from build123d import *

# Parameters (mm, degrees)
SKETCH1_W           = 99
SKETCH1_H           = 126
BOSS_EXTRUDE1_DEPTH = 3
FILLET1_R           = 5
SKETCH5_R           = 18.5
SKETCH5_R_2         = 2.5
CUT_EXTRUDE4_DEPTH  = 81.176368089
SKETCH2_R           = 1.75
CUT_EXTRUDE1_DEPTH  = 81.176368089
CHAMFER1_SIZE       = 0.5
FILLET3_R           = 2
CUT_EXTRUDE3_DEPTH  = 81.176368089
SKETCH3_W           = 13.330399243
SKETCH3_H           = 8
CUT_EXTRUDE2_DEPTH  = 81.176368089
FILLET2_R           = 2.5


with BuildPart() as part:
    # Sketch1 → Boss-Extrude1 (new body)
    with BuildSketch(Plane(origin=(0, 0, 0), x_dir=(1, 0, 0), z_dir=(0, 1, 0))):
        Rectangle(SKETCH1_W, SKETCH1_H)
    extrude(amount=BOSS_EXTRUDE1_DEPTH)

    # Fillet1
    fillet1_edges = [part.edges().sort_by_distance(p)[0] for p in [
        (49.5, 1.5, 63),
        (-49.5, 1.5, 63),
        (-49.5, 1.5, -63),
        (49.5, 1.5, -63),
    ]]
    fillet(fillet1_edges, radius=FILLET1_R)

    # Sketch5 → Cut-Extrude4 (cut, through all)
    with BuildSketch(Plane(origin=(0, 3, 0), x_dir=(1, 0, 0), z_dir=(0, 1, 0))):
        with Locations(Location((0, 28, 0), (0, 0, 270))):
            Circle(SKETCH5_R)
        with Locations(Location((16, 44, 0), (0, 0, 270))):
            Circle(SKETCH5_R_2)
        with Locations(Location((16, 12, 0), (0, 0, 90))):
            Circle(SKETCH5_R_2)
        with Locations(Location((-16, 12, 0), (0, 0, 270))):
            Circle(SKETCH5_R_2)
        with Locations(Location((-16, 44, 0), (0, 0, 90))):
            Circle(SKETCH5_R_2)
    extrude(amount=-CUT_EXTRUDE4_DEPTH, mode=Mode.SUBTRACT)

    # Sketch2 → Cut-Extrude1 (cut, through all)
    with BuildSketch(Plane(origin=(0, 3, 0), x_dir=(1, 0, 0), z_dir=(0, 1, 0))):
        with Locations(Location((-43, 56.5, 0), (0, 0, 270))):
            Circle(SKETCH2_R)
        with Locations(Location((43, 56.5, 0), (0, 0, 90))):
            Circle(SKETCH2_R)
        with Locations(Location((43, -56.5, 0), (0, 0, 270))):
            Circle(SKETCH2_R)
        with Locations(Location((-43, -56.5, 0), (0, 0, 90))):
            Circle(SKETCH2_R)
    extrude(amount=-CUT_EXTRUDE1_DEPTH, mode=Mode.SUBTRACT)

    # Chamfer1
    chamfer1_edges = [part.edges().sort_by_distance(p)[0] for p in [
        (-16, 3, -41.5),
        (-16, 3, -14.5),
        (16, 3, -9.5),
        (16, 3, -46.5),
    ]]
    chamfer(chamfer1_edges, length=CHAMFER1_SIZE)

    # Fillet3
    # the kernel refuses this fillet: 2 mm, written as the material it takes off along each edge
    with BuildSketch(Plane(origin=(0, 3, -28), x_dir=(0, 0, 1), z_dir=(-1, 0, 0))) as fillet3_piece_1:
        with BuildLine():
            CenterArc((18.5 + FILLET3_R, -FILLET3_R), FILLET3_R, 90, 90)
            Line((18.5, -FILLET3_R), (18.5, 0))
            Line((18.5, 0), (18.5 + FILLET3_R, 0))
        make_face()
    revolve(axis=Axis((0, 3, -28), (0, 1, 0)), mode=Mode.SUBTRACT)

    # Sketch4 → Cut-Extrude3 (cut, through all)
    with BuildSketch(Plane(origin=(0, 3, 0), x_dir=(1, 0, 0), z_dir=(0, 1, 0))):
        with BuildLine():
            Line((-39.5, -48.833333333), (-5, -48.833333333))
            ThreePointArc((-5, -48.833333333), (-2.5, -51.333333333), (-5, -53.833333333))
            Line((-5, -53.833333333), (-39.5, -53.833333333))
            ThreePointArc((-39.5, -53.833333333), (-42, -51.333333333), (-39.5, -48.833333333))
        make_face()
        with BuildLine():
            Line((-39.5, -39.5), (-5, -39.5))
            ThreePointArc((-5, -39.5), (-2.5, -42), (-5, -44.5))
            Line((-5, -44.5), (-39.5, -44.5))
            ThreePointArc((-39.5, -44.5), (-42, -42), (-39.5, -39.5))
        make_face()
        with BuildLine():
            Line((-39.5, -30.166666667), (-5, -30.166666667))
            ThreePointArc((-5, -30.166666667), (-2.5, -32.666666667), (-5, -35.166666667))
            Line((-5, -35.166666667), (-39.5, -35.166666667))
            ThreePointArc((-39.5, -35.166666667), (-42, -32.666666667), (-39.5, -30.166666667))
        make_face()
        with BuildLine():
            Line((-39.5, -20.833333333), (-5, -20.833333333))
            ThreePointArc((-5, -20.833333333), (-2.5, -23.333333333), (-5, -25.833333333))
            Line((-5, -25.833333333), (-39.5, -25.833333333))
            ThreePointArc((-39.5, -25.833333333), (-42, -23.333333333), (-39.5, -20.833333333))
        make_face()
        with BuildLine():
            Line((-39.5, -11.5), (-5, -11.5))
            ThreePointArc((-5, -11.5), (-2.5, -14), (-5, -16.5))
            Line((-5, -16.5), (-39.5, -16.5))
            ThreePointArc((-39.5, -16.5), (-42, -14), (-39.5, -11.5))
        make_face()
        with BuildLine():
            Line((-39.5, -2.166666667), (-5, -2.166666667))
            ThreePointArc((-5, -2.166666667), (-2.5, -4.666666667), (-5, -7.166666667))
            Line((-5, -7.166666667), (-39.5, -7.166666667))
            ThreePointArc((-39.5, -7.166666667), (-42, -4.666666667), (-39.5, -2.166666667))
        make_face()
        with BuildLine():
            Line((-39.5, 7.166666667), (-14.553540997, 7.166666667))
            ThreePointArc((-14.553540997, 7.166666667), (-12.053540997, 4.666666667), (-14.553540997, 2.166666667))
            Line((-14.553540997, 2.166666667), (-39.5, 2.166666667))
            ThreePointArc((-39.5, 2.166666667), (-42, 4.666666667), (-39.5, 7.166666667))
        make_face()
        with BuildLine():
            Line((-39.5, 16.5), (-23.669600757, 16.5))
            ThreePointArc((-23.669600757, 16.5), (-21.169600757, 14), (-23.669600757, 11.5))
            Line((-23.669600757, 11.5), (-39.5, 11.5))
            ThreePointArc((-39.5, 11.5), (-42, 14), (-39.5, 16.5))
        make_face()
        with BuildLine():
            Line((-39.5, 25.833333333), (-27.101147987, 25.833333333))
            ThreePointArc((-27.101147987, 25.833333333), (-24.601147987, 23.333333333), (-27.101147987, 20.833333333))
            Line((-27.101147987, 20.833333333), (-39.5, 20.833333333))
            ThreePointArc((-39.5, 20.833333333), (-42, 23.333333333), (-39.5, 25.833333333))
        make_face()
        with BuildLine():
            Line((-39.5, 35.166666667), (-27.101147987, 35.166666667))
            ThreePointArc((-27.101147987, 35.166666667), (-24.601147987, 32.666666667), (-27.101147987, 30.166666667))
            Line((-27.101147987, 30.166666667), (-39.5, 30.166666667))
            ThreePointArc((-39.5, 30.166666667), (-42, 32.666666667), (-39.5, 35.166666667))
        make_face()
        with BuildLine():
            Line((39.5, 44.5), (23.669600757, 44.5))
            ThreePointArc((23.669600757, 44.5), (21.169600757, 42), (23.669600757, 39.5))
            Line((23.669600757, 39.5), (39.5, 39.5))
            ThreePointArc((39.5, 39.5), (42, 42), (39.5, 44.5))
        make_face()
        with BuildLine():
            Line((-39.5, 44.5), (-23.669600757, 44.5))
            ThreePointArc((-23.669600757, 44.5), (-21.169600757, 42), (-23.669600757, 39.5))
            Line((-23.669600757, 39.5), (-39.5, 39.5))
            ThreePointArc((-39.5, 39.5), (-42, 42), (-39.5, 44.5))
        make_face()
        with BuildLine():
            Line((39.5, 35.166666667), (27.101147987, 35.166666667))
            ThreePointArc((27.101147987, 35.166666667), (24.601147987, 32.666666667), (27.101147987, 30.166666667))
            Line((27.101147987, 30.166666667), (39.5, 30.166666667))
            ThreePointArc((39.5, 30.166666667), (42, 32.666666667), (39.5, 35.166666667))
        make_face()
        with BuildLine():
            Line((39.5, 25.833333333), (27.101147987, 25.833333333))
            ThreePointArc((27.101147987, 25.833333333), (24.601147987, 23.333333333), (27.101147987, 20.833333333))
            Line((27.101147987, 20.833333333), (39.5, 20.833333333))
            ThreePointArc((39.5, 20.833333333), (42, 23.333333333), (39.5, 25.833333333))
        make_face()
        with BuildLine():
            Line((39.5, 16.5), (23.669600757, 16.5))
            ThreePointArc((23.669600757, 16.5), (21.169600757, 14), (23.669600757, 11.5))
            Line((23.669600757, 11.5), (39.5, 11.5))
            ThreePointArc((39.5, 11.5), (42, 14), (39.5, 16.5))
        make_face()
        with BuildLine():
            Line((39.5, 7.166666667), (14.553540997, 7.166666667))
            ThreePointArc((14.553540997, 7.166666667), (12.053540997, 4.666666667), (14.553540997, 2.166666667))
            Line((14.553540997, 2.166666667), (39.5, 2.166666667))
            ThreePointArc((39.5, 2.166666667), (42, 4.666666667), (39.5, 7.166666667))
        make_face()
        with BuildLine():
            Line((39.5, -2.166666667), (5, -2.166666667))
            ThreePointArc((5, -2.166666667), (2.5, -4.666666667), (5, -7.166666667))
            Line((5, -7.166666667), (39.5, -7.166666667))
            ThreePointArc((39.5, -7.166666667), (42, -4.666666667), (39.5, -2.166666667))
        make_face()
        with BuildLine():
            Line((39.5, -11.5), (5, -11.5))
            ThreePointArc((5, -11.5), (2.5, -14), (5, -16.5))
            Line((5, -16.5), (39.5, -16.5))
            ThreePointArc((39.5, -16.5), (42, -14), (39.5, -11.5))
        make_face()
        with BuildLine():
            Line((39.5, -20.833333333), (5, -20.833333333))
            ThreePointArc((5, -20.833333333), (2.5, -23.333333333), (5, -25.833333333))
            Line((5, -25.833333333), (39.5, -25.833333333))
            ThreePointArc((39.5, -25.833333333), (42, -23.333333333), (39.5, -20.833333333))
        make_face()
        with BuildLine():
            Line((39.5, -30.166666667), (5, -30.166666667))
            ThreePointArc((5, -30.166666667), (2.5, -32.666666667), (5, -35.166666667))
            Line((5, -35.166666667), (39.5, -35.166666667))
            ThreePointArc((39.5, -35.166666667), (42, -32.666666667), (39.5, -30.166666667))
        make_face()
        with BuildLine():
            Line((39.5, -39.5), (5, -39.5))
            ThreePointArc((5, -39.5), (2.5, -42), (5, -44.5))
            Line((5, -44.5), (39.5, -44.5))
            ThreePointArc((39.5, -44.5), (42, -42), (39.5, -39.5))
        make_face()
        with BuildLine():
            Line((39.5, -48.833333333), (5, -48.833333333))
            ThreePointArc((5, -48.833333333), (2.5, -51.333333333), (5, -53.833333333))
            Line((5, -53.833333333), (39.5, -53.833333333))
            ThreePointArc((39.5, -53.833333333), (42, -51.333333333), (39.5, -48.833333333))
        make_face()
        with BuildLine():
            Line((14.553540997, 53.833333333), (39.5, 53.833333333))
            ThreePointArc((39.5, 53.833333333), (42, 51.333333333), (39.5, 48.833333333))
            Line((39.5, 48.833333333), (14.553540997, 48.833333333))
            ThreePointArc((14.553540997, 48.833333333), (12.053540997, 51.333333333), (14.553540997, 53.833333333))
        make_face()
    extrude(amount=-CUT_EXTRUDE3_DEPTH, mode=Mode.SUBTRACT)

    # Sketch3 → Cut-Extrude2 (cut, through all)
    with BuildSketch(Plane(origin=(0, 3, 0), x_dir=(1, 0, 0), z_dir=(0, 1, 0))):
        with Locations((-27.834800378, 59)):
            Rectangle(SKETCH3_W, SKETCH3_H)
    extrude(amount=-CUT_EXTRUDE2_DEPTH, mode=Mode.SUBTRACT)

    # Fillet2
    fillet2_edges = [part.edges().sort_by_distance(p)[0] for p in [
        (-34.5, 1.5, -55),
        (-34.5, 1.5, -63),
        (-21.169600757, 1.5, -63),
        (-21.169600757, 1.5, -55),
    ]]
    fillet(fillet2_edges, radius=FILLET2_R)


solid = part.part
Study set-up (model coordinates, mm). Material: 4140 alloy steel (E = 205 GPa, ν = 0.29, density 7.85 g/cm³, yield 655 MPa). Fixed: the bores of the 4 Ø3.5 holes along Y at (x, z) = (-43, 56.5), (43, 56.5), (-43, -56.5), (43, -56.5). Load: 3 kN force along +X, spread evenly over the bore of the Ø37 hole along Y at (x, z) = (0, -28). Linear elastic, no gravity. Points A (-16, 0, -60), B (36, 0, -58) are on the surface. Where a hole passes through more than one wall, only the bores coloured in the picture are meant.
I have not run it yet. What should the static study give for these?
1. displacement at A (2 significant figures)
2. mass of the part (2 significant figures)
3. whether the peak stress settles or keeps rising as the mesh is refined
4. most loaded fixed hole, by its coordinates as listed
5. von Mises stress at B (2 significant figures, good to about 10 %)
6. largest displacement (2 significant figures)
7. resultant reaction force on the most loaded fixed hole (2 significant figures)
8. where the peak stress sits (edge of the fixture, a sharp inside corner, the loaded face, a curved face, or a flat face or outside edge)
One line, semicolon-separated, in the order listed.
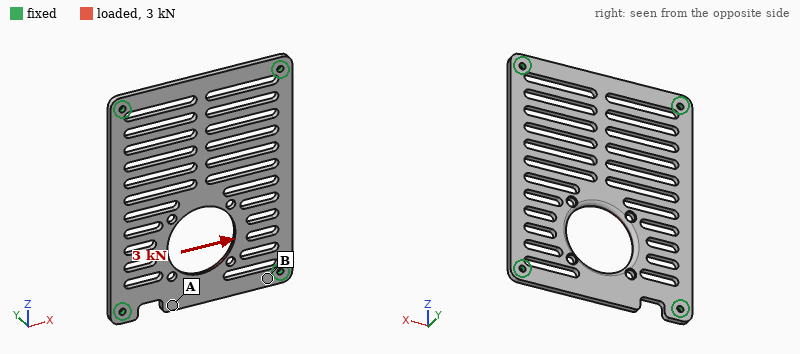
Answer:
8.5 µm; 180 g; keeps rising; (43, -56.5); 37 MPa; 43 µm; 1.6 kN; a sharp inside corner
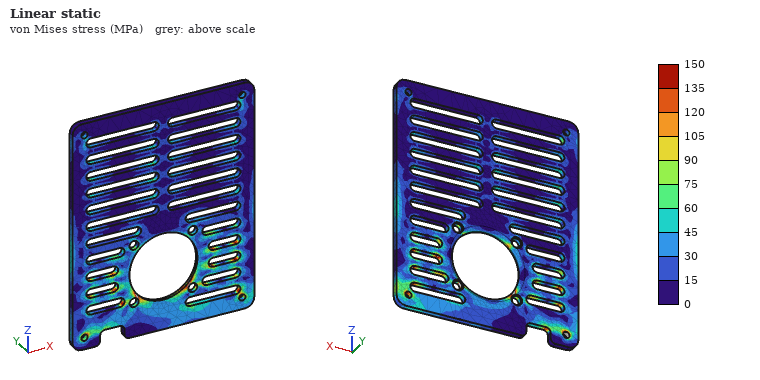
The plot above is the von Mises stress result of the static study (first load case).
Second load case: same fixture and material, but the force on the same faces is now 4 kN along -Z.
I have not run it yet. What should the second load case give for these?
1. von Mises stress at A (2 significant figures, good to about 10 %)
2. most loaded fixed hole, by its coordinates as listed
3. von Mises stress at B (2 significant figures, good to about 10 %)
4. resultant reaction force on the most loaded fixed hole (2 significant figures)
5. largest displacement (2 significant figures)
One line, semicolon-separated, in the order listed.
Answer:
29 MPa; (-43, -56.5); 57 MPa; 1.7 kN; 79 µm
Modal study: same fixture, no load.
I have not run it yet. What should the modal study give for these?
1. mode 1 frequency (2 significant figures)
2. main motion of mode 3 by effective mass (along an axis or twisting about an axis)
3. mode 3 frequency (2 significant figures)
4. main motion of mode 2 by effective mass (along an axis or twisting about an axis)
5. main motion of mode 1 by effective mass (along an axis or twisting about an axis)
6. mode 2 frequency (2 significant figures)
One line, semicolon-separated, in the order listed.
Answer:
740 Hz; twisting about X; 1700 Hz; twisting about Z; along Y; 1200 Hz
